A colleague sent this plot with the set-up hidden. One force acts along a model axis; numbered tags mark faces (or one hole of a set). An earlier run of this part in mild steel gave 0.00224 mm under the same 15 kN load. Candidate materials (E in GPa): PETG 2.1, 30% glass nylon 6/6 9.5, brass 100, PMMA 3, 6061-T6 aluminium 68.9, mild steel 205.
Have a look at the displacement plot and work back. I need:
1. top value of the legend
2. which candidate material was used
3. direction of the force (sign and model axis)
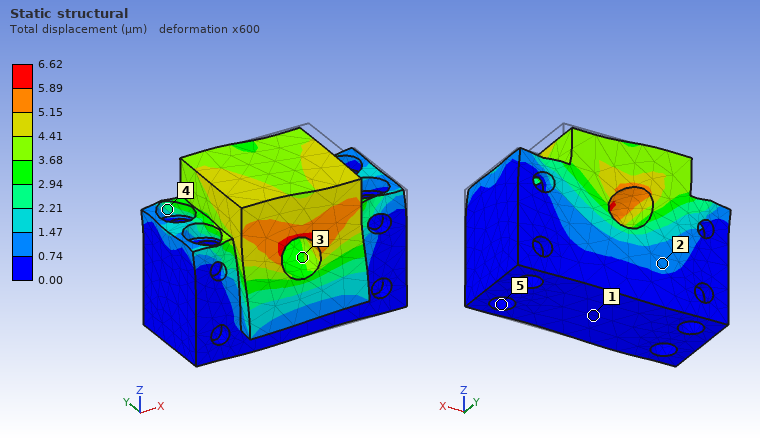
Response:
6.62 µm
6061-T6 aluminium
-X
